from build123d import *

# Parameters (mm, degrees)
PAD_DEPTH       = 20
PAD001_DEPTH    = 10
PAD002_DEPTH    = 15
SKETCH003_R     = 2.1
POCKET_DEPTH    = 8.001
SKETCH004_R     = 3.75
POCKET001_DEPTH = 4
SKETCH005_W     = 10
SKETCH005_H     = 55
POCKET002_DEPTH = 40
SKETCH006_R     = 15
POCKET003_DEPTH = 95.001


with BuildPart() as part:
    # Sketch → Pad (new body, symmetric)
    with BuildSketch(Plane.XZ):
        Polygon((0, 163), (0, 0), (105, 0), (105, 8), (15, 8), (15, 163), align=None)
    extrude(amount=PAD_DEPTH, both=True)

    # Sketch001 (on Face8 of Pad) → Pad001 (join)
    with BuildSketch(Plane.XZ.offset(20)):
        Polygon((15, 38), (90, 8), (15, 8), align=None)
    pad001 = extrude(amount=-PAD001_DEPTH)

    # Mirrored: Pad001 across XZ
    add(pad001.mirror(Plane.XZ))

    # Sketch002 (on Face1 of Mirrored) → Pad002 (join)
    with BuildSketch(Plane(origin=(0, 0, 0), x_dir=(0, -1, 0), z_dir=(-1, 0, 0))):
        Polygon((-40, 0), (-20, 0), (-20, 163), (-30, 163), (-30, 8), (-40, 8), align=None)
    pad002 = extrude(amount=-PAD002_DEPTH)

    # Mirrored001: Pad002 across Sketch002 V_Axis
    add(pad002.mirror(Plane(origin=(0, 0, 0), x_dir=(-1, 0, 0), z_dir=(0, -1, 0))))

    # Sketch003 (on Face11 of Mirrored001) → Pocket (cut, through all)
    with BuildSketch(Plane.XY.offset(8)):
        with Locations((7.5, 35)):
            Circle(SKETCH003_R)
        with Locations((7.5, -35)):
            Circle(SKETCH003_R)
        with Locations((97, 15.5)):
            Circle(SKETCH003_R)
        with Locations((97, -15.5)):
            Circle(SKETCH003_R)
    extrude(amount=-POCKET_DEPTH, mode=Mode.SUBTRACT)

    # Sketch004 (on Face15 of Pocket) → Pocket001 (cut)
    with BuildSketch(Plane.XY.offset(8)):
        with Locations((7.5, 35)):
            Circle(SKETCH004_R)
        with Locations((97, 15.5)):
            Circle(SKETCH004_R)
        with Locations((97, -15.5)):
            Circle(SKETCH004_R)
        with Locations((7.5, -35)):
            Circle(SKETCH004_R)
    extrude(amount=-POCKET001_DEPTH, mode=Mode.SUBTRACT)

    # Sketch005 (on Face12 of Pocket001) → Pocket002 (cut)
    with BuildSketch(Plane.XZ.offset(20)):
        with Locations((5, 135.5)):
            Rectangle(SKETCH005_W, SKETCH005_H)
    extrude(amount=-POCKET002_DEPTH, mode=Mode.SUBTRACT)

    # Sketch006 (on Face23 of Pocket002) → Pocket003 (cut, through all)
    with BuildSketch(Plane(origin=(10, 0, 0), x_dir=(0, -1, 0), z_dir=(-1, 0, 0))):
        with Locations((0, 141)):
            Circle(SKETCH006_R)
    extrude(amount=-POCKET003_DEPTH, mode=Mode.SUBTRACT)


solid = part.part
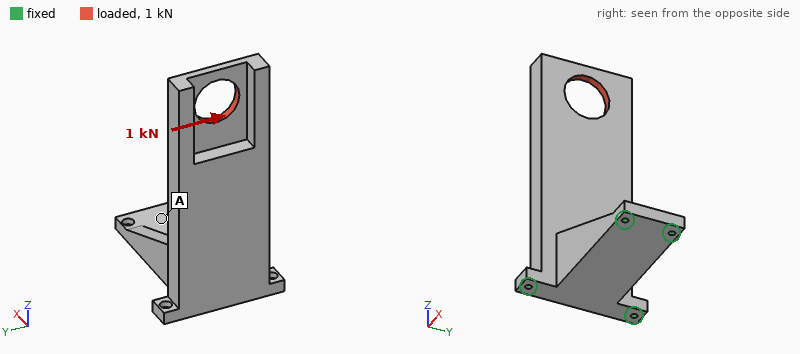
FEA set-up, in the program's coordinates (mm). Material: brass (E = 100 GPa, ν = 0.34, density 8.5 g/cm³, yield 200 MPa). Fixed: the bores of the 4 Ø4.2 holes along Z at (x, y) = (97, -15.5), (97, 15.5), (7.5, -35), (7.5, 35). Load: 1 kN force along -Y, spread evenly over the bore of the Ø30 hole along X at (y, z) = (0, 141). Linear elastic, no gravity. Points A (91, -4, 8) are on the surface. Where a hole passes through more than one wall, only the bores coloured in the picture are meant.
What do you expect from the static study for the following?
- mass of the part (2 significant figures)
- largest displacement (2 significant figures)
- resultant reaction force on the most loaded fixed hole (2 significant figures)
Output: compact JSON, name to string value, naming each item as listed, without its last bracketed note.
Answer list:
{"mass of the part": "1.5 kg", "largest displacement": "0.10 mm", "resultant reaction force on the most loaded fixed hole": "2.1 kN"}
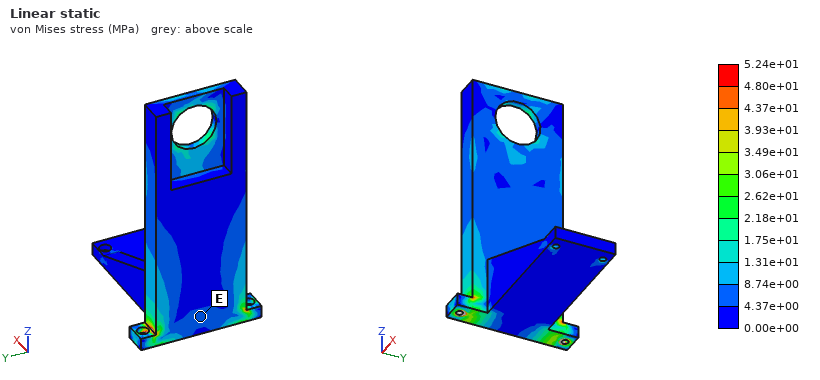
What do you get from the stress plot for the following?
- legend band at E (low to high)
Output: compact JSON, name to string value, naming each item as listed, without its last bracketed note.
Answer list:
{"legend band at E": "4.37e+00 to 8.74e+00 MPa"}
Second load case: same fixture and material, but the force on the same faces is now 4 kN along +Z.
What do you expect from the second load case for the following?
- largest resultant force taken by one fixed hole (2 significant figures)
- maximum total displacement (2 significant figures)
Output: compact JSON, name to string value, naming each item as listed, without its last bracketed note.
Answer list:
{"largest resultant force taken by one fixed hole": "2.2 kN", "maximum total displacement": "0.11 mm"}
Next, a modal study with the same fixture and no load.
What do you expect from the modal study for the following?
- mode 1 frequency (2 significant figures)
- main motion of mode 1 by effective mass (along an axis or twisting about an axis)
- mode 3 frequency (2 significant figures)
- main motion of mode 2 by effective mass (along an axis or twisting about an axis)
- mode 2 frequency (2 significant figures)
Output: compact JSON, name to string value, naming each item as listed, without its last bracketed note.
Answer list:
{"mode 1 frequency": "510 Hz", "main motion of mode 1 by effective mass": "along X", "mode 3 frequency": "1500 Hz", "main motion of mode 2 by effective mass": "along Y", "mode 2 frequency": "1000 Hz"}
